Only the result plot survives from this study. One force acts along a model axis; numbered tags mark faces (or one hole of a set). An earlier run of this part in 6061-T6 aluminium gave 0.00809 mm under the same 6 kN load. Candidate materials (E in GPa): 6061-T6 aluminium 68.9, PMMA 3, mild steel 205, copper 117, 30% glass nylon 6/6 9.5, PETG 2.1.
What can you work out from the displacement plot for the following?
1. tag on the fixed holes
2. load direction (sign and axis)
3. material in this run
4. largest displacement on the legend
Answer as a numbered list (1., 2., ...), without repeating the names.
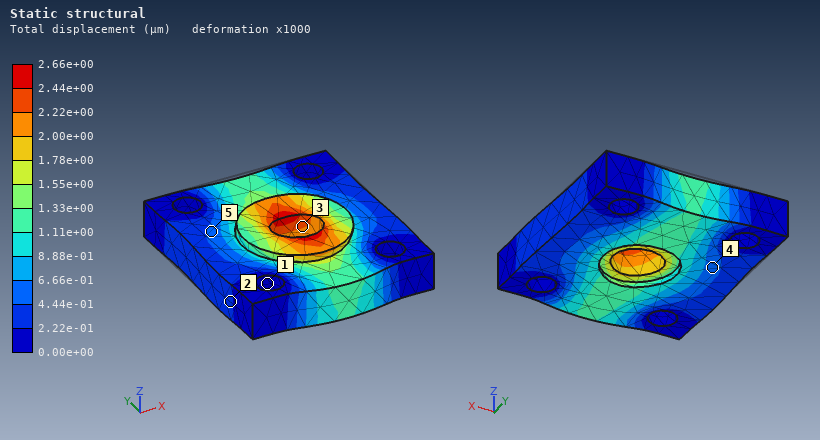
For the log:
1. 1
2. -Y
3. mild steel
4. 2.66e+00 µm
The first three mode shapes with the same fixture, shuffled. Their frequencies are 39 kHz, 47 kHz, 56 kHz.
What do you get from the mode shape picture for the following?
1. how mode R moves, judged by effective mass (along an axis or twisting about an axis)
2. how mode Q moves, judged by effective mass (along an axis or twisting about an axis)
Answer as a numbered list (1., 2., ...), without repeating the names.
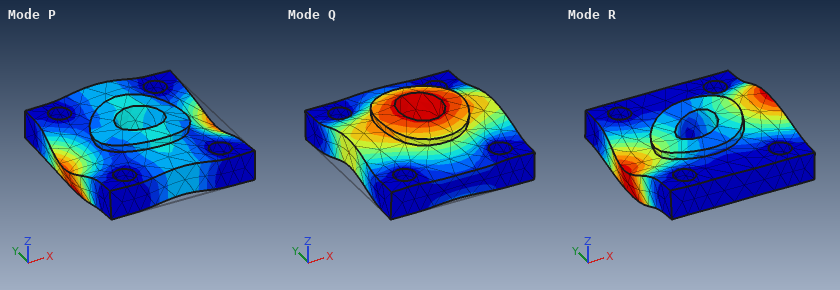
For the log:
1. twisting about Y
2. along Z
